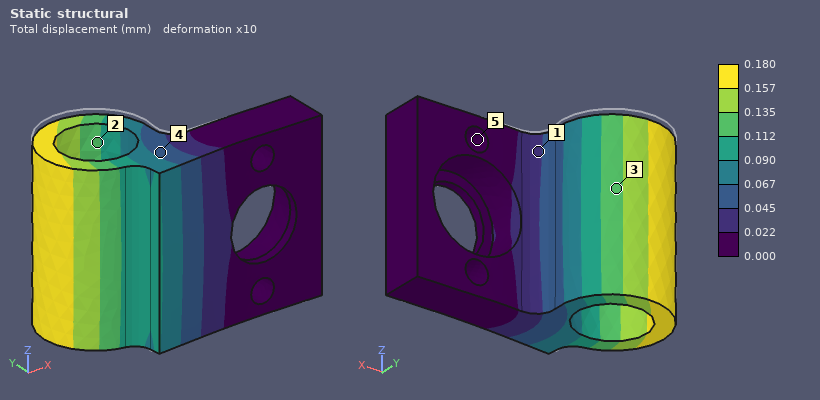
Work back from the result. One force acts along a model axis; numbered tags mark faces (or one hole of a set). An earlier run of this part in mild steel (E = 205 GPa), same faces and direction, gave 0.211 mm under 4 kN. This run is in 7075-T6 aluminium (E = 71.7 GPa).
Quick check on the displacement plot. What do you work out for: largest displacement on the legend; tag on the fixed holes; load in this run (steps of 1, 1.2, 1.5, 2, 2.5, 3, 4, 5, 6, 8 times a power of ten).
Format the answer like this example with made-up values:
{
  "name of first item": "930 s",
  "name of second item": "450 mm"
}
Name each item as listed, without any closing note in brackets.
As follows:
{
  "largest displacement on the legend": "0.180 mm",
  "tag on the fixed holes": "5",
  "load in this run": "1.2 kN"
}
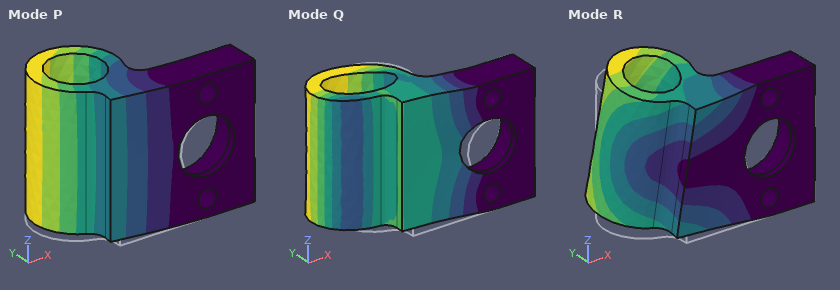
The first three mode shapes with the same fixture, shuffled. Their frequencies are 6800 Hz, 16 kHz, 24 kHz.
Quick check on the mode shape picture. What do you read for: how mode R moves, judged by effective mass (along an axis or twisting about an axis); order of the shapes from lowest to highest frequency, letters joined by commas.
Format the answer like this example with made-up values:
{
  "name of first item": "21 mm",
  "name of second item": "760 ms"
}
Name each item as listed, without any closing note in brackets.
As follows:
{
  "how mode R moves, judged by effective mass": "along Z",
  "order of the shapes from lowest to highest frequency, letters joined by commas": "P, R, Q"
}
